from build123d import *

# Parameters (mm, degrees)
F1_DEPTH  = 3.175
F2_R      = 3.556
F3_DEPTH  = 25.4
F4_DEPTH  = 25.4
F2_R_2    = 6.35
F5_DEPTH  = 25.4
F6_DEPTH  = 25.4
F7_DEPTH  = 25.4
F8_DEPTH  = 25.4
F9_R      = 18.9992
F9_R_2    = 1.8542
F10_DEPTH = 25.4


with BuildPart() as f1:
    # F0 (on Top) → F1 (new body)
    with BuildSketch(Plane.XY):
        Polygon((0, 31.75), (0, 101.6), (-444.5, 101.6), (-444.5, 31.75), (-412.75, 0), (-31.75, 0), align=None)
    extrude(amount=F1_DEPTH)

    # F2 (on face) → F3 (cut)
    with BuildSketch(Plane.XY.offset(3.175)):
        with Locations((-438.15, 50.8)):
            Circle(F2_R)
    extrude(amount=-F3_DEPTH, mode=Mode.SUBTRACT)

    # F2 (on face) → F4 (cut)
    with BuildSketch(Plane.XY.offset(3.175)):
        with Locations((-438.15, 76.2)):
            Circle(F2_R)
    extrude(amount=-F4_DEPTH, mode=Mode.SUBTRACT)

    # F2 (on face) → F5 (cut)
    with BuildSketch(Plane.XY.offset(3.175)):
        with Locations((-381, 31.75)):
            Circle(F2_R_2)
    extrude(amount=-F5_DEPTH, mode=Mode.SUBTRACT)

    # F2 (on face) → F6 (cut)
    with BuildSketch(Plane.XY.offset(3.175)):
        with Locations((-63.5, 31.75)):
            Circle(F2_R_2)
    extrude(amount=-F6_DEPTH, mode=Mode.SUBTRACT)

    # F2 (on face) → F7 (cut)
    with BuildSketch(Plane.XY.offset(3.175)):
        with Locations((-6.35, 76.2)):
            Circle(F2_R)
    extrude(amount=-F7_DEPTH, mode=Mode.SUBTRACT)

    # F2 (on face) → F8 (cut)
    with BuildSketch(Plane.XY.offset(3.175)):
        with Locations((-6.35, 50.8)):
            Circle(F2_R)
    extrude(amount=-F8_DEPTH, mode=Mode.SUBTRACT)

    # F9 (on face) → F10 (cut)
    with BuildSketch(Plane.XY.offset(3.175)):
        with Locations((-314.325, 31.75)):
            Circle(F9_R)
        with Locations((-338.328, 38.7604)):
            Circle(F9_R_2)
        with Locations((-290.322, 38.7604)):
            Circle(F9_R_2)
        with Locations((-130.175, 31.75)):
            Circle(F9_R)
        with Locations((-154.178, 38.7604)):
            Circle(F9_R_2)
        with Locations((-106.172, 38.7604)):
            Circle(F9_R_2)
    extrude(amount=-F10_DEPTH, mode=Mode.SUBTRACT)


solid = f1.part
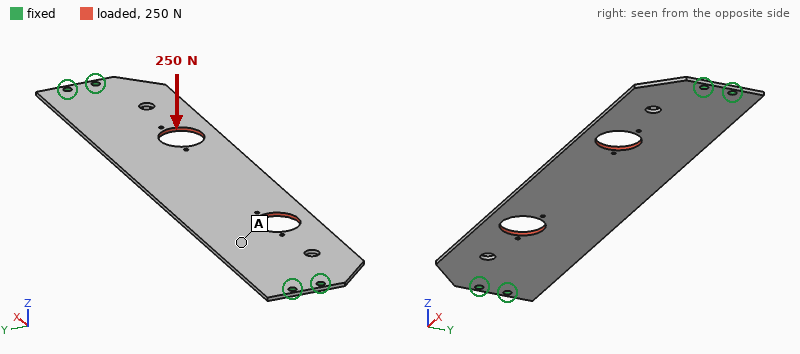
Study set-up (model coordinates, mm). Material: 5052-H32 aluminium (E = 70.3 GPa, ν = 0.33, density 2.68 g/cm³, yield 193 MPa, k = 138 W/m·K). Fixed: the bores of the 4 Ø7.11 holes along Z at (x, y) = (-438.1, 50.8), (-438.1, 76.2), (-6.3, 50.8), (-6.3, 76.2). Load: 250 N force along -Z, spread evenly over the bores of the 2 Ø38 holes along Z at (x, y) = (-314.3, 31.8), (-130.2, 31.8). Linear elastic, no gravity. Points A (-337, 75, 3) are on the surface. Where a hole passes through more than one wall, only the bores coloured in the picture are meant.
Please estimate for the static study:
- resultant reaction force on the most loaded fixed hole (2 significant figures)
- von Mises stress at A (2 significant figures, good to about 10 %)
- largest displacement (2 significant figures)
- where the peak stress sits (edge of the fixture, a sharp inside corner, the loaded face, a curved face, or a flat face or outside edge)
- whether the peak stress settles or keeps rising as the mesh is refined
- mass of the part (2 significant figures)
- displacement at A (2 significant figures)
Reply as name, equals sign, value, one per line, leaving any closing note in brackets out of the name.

resultant reaction force on the most loaded fixed hole = 170 N
von Mises stress at A = 18 MPa
largest displacement = 4.6 mm
where the peak stress sits = edge of the fixture
whether the peak stress settles or keeps rising as the mesh is refined = keeps rising
mass of the part = 350 g
displacement at A = 1.9 mm
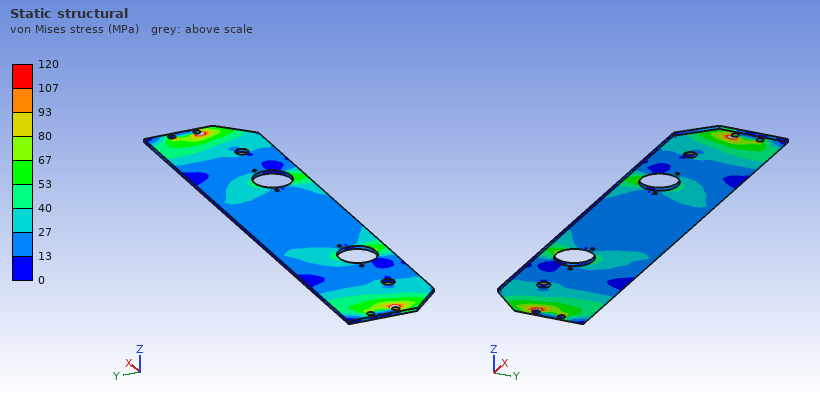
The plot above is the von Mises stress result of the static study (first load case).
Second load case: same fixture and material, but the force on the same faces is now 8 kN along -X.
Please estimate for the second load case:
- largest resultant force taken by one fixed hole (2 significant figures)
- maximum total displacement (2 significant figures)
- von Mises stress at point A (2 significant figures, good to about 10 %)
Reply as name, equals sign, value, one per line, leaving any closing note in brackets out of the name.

largest resultant force taken by one fixed hole = 2.2 kN
maximum total displacement = 42 µm
von Mises stress at point A = 13 MPa
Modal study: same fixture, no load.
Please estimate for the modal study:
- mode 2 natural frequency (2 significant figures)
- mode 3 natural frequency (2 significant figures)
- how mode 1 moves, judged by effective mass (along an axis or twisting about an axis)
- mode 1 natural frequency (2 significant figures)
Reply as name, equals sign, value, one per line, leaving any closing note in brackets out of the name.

mode 2 natural frequency = 230 Hz
mode 3 natural frequency = 240 Hz
how mode 1 moves, judged by effective mass = along Z
mode 1 natural frequency = 88 Hz
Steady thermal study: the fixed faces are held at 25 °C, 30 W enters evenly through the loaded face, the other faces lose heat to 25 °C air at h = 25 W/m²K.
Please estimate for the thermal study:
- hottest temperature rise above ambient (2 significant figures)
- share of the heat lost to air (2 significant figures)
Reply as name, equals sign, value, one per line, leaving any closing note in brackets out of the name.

hottest temperature rise above ambient = 22 K
share of the heat lost to air = 74 %
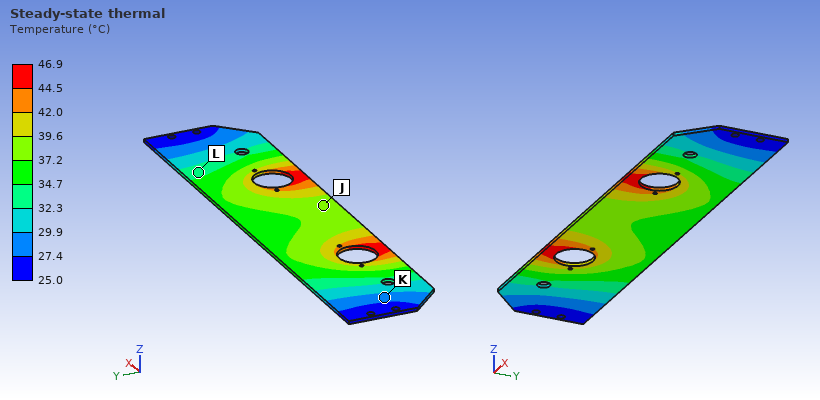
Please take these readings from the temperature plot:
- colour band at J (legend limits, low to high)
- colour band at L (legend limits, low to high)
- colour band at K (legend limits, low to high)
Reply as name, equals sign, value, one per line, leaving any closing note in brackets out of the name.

colour band at J = 37.2 to 39.6 °C
colour band at L = 32.3 to 34.7 °C
colour band at K = 27.4 to 29.9 °C
